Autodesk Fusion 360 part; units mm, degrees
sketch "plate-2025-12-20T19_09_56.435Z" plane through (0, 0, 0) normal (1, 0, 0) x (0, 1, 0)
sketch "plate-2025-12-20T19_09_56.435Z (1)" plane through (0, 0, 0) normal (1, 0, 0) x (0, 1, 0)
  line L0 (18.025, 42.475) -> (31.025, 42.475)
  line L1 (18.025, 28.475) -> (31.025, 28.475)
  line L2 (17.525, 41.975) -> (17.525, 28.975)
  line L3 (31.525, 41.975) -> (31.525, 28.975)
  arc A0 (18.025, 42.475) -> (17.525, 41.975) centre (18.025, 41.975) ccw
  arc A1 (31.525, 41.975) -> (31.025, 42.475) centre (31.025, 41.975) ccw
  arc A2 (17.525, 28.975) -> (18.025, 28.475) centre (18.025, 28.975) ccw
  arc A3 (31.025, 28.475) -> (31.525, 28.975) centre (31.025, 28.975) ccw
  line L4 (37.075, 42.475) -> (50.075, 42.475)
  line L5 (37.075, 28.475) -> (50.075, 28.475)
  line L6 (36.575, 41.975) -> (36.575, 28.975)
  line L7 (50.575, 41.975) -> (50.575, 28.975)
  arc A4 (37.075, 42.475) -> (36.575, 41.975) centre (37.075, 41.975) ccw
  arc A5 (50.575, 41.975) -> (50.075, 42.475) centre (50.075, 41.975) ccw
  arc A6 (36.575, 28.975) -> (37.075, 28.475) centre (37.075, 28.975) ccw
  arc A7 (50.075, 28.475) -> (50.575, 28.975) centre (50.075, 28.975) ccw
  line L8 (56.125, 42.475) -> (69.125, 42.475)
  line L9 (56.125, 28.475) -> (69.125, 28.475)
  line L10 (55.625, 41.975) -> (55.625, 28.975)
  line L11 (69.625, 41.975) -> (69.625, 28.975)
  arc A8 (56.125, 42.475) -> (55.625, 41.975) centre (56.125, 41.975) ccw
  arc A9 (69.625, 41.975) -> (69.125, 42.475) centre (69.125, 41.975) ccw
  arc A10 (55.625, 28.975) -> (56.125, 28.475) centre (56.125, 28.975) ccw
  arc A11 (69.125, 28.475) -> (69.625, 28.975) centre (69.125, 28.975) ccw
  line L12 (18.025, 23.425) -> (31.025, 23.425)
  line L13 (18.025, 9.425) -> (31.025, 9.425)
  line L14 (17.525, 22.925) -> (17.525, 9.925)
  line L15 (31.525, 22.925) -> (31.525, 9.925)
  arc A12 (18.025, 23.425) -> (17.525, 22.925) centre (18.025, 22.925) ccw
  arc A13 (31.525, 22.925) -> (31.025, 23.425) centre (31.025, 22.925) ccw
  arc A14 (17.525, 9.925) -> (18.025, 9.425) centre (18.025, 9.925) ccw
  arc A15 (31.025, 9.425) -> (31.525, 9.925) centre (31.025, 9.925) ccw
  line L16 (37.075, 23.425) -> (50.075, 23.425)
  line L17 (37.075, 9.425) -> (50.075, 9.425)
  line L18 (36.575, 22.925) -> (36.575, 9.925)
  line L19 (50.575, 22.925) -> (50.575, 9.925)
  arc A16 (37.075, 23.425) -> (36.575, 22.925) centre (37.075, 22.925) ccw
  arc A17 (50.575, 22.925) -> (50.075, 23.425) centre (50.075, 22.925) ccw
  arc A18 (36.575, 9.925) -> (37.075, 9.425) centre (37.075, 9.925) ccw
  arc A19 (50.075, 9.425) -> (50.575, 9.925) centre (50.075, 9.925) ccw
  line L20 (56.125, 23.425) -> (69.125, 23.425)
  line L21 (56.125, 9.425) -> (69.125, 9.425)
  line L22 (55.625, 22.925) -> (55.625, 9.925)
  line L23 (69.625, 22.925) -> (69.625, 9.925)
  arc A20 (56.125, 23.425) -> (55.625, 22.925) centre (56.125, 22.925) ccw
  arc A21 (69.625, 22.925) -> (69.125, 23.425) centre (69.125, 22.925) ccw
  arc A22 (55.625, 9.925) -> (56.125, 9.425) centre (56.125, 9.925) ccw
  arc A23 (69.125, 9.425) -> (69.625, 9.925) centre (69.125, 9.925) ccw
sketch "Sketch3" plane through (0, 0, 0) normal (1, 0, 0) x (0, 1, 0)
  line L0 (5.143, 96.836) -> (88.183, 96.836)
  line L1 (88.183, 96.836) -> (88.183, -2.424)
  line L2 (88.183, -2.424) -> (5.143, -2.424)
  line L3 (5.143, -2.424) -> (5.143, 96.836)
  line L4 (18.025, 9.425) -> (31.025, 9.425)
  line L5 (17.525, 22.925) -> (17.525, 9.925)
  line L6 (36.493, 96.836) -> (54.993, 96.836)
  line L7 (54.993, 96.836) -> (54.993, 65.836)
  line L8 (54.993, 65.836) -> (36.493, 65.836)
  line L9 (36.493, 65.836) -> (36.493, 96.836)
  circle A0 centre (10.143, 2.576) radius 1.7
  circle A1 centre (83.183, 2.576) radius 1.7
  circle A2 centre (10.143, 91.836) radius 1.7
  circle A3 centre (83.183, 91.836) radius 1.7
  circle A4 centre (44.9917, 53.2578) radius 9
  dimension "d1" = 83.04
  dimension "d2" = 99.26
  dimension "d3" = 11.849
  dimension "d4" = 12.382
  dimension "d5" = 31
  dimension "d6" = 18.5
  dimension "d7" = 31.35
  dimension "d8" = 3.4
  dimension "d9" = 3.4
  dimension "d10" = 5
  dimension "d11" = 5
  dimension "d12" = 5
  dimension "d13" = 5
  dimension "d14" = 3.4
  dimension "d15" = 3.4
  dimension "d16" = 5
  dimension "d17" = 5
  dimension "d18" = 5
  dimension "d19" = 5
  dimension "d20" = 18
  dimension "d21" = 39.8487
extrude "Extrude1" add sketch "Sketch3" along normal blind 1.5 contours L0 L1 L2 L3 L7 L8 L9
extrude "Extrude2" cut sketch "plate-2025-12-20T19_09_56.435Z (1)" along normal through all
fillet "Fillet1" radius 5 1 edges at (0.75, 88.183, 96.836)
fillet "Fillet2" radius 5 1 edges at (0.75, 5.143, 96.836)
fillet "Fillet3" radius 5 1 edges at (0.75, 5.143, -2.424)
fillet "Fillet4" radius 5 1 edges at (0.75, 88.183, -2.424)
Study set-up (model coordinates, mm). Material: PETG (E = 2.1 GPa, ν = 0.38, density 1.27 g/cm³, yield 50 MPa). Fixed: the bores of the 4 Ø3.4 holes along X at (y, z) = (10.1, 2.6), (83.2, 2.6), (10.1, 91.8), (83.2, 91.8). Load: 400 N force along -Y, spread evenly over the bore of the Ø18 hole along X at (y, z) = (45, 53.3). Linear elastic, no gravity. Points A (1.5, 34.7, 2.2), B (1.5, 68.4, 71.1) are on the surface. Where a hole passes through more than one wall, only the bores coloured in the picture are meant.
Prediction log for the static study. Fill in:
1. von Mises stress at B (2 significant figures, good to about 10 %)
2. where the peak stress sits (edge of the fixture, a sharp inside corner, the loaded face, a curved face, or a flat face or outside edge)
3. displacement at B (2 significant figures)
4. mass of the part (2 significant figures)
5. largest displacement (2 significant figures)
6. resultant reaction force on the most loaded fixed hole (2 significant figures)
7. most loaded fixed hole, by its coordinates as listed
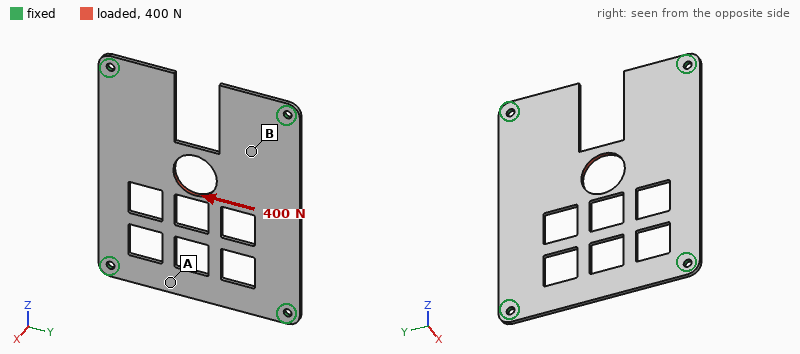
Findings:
7.3 MPa
a curved face
0.28 mm
12 g
0.54 mm
190 N
(83.2, 91.8)
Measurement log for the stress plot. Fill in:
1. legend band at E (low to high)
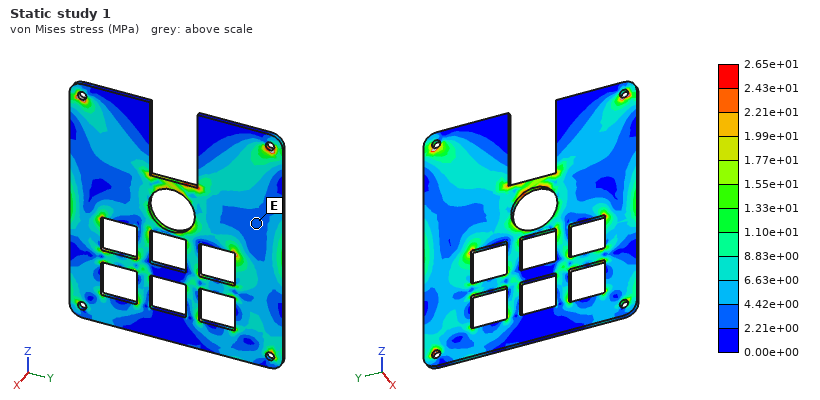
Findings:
2.21e+00 to 4.42e+00 MPa
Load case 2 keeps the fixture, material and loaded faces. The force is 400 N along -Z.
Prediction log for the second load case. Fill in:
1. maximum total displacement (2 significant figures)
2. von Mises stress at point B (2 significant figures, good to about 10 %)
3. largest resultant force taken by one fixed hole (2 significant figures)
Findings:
0.37 mm
5.0 MPa
160 N
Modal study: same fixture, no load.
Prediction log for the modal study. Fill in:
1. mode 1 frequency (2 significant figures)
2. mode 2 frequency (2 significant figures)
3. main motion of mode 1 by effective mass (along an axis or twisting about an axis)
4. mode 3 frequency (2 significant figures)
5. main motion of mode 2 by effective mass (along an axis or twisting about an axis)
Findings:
190 Hz
280 Hz
along X
360 Hz
twisting about Z
